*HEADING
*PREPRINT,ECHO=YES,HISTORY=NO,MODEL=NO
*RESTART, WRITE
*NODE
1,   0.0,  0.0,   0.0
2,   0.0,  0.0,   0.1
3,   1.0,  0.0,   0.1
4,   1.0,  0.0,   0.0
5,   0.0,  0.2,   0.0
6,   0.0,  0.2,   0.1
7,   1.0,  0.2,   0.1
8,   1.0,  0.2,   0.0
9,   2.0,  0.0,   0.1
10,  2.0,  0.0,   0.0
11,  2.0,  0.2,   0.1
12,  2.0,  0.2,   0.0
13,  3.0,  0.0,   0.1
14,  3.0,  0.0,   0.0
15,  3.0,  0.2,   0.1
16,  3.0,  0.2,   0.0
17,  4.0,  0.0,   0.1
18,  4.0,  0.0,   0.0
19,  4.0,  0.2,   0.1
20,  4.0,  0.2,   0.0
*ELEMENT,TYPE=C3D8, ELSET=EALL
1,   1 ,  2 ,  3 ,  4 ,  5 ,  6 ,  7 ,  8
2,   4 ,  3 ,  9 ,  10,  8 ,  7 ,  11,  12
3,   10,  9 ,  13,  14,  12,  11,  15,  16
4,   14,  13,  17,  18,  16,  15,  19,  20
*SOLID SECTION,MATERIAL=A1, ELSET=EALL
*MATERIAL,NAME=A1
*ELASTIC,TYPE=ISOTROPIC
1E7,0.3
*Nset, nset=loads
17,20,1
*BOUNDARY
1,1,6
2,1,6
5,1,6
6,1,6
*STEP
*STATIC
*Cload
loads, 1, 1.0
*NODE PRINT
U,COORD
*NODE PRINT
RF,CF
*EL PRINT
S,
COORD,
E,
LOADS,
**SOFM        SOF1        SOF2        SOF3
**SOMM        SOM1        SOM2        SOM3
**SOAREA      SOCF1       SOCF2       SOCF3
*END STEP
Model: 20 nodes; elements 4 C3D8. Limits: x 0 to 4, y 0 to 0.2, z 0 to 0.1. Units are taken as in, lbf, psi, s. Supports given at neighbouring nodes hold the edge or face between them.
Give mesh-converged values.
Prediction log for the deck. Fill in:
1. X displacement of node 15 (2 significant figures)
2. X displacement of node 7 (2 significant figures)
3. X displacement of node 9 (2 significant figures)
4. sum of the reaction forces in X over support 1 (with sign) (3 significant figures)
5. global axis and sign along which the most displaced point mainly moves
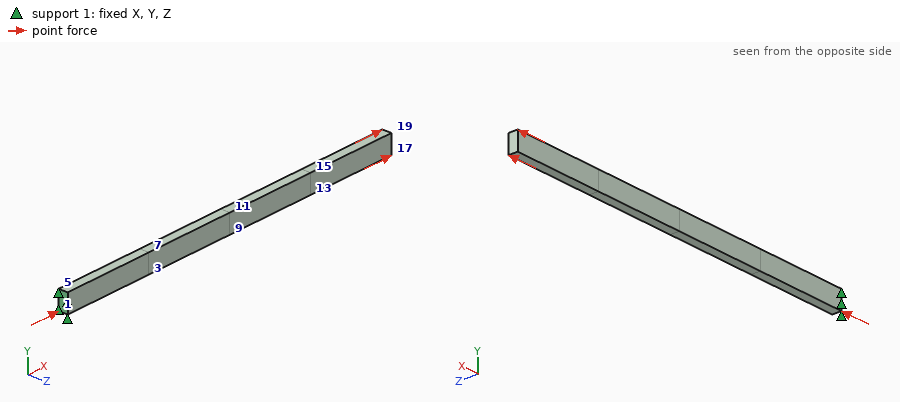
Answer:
3.0e-05 in
9.8e-06 in
2.0e-05 in
-3.00 lbf
+X
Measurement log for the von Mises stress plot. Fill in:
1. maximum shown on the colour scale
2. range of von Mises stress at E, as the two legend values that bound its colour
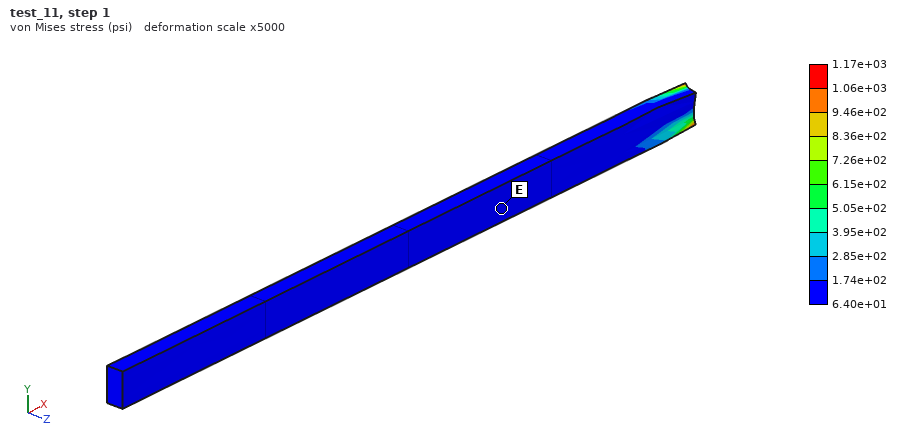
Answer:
1.17e+03 psi
6.40e+01 to 1.74e+02 psi
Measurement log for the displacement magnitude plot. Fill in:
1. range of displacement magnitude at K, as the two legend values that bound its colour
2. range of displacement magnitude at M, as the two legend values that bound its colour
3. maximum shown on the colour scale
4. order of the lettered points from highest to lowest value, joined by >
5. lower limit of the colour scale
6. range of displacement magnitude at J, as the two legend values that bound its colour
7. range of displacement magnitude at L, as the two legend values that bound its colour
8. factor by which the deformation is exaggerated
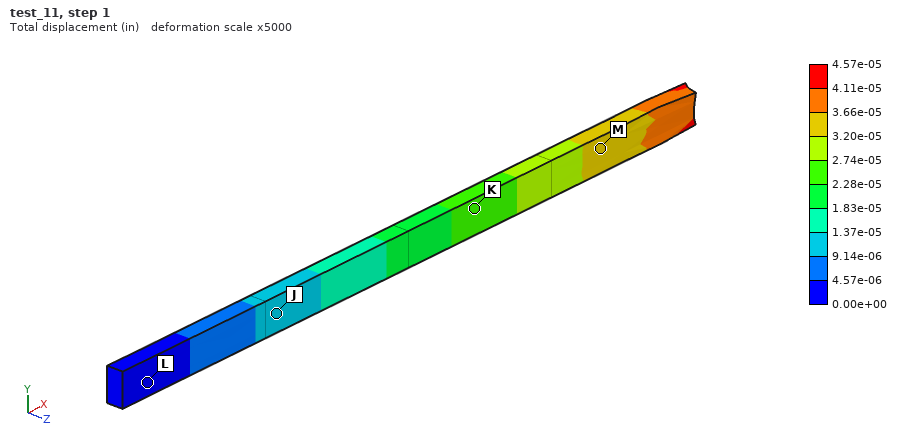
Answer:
2.28e-05 to 2.74e-05 in
3.20e-05 to 3.66e-05 in
4.57e-05 in
M > K > J > L
0.00e+00 in
9.14e-06 to 1.37e-05 in
0.00e+00 to 4.57e-06 in
5000
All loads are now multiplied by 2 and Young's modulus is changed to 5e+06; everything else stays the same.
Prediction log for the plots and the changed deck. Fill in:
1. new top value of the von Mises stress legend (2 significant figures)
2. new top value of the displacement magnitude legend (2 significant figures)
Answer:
2300 psi
1.8e-04 in
